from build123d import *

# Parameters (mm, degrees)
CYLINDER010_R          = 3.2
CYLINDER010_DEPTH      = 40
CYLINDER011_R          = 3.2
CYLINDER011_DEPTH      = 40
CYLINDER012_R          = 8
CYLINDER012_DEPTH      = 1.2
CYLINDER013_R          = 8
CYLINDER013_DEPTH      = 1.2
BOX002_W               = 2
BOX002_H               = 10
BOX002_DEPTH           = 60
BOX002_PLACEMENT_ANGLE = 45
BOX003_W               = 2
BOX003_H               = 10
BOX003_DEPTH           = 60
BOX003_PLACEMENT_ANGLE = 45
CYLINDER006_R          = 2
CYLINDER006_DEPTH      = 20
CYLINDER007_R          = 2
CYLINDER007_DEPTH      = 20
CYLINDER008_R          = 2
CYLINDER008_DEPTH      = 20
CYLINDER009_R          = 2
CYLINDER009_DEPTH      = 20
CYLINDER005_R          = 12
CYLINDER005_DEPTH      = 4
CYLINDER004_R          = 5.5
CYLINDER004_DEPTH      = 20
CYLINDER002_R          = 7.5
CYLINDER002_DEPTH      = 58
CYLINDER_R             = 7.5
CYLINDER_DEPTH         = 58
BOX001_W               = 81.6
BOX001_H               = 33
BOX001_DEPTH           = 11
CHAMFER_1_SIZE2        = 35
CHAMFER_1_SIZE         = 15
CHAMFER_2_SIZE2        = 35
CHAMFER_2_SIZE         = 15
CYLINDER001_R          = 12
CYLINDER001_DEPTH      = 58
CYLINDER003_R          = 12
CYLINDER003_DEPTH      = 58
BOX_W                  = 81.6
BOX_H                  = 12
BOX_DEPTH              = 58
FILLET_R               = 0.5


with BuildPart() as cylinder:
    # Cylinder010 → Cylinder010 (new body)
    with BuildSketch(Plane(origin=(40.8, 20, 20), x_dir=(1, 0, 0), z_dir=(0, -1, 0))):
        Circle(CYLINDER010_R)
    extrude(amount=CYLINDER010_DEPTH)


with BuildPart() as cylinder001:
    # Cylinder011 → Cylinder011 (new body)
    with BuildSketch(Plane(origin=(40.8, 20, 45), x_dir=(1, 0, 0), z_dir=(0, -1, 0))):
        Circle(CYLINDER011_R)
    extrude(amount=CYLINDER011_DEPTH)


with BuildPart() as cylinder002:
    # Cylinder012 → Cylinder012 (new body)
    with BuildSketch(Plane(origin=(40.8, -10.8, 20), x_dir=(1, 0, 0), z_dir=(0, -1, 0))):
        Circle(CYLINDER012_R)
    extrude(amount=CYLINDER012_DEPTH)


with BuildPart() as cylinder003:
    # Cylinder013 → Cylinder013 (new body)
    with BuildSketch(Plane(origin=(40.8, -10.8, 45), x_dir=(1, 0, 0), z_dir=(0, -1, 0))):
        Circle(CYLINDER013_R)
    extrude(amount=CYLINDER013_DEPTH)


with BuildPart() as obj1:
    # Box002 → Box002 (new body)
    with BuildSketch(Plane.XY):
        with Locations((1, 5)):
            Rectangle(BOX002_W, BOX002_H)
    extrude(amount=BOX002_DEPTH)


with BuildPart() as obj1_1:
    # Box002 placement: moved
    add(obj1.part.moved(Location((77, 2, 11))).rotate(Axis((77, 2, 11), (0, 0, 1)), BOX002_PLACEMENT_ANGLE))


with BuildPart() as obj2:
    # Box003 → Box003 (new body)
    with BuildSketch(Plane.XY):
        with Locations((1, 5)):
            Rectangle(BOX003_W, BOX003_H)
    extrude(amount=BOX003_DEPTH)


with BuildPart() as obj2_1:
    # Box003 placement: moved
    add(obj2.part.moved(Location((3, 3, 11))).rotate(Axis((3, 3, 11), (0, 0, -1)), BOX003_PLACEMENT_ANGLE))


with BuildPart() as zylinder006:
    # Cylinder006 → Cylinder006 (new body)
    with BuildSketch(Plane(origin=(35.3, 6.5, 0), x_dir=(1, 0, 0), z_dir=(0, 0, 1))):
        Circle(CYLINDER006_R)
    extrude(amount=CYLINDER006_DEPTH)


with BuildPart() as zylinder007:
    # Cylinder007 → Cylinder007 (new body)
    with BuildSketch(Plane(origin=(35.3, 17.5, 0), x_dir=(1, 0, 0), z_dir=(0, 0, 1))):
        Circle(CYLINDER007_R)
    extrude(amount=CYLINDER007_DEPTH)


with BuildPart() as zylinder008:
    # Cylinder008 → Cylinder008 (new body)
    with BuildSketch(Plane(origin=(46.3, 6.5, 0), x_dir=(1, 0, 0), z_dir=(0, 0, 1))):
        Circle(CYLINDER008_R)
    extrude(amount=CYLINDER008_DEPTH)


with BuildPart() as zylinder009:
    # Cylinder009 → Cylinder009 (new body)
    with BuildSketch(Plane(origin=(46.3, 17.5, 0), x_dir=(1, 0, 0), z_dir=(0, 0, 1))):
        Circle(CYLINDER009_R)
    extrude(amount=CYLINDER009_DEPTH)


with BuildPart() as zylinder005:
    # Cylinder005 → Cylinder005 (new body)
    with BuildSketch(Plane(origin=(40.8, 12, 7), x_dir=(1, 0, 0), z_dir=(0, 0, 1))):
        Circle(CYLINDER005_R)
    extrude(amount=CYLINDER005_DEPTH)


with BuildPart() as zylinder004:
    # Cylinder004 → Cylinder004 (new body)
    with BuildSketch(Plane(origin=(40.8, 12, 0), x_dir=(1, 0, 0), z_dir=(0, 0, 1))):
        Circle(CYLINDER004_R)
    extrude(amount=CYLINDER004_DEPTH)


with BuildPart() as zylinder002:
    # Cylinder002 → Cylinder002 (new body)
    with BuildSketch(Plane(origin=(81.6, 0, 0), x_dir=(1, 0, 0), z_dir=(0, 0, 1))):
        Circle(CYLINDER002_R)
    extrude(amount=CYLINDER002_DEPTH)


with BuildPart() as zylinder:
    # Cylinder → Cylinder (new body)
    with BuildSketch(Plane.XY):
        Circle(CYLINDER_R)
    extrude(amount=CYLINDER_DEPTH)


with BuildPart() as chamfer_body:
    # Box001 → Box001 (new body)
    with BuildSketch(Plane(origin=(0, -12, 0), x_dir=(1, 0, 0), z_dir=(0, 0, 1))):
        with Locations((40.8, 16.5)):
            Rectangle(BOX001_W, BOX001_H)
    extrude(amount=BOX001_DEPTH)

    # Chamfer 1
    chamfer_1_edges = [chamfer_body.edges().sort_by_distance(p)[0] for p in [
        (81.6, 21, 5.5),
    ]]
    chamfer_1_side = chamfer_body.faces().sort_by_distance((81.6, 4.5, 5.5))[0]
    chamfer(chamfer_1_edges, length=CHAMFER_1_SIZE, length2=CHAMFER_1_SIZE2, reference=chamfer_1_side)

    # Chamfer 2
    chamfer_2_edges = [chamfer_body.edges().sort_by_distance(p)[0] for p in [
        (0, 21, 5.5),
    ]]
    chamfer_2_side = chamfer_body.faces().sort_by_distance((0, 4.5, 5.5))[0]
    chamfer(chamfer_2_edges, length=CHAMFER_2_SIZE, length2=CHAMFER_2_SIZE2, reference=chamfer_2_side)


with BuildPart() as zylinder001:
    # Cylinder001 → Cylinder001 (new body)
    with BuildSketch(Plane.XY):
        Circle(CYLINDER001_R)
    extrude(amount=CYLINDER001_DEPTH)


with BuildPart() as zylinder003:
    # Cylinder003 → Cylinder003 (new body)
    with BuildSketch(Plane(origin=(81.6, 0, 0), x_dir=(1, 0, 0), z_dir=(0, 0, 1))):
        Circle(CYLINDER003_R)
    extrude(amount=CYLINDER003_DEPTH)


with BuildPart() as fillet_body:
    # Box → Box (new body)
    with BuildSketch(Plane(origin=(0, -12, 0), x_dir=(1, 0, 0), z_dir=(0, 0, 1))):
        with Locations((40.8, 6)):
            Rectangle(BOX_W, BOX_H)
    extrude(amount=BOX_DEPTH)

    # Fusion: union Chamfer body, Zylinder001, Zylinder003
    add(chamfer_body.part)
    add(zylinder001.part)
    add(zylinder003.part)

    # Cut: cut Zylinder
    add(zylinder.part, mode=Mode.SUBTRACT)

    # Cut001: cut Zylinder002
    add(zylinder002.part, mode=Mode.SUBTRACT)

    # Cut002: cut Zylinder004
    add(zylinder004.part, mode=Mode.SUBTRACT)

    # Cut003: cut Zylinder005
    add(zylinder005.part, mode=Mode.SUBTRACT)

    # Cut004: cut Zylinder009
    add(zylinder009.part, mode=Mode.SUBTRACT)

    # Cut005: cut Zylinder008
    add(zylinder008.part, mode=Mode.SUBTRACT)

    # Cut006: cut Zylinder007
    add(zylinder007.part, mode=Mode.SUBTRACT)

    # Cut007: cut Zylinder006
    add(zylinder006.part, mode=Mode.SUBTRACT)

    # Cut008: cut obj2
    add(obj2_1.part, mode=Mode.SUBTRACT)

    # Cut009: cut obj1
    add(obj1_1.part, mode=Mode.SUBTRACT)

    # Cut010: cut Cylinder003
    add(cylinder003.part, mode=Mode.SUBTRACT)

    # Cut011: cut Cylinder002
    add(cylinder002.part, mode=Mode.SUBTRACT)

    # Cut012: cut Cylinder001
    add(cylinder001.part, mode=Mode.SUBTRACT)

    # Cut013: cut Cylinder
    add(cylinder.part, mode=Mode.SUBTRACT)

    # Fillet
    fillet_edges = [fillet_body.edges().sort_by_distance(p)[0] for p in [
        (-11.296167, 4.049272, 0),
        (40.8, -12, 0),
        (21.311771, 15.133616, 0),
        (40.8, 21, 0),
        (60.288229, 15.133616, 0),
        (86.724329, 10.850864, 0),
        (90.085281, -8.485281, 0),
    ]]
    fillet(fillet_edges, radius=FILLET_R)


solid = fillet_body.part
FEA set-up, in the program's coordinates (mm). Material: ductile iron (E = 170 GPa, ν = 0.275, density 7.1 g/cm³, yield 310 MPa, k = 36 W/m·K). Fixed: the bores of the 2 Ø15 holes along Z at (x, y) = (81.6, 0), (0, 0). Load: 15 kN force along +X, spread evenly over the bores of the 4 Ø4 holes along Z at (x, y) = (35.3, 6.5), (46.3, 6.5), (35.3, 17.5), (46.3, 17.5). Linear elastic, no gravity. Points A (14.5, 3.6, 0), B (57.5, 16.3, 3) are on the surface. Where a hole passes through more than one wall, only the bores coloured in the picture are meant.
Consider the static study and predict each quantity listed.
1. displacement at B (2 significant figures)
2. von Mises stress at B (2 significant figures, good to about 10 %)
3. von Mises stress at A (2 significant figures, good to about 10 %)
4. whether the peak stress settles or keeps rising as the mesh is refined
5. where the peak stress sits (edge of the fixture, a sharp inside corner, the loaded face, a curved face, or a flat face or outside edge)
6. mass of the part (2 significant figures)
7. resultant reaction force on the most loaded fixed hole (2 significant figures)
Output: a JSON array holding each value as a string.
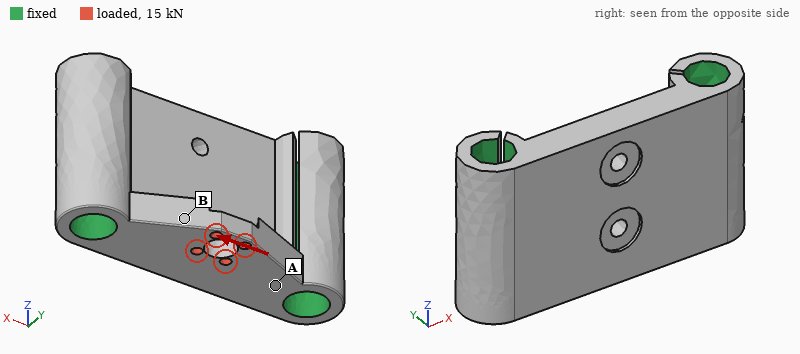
["8.4 µm", "94 MPa", "38 MPa", "keeps rising", "a sharp inside corner", "580 g", "8.1 kN"]
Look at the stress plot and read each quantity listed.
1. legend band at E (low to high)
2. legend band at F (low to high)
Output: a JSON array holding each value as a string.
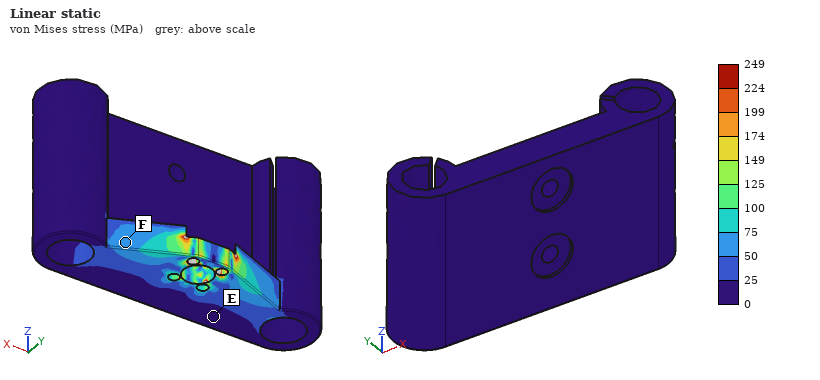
["0 to 25 MPa", "50 to 75 MPa"]
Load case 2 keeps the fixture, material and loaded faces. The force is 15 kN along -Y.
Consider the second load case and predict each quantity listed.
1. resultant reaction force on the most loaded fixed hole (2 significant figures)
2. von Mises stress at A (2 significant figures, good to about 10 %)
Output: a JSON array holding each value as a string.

["7.5 kN", "91 MPa"]
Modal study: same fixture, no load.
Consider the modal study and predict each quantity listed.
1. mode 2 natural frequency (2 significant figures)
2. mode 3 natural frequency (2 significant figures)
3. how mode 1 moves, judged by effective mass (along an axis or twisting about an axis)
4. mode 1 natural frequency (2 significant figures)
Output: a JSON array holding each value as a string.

["13 kHz", "16 kHz", "along Y", "12 kHz"]
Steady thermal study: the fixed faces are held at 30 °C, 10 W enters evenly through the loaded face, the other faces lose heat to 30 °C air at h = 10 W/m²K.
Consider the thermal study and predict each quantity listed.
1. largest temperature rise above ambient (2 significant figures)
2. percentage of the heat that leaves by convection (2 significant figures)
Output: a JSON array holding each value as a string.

["29 K", "4.6 %"]
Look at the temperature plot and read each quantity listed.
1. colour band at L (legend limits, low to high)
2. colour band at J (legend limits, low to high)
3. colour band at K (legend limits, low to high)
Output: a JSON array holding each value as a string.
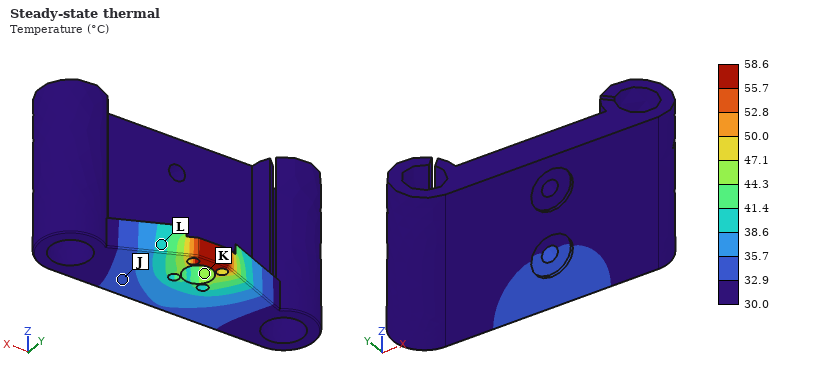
["38.6 to 41.4 °C", "32.9 to 35.7 °C", "44.3 to 47.1 °C"]
